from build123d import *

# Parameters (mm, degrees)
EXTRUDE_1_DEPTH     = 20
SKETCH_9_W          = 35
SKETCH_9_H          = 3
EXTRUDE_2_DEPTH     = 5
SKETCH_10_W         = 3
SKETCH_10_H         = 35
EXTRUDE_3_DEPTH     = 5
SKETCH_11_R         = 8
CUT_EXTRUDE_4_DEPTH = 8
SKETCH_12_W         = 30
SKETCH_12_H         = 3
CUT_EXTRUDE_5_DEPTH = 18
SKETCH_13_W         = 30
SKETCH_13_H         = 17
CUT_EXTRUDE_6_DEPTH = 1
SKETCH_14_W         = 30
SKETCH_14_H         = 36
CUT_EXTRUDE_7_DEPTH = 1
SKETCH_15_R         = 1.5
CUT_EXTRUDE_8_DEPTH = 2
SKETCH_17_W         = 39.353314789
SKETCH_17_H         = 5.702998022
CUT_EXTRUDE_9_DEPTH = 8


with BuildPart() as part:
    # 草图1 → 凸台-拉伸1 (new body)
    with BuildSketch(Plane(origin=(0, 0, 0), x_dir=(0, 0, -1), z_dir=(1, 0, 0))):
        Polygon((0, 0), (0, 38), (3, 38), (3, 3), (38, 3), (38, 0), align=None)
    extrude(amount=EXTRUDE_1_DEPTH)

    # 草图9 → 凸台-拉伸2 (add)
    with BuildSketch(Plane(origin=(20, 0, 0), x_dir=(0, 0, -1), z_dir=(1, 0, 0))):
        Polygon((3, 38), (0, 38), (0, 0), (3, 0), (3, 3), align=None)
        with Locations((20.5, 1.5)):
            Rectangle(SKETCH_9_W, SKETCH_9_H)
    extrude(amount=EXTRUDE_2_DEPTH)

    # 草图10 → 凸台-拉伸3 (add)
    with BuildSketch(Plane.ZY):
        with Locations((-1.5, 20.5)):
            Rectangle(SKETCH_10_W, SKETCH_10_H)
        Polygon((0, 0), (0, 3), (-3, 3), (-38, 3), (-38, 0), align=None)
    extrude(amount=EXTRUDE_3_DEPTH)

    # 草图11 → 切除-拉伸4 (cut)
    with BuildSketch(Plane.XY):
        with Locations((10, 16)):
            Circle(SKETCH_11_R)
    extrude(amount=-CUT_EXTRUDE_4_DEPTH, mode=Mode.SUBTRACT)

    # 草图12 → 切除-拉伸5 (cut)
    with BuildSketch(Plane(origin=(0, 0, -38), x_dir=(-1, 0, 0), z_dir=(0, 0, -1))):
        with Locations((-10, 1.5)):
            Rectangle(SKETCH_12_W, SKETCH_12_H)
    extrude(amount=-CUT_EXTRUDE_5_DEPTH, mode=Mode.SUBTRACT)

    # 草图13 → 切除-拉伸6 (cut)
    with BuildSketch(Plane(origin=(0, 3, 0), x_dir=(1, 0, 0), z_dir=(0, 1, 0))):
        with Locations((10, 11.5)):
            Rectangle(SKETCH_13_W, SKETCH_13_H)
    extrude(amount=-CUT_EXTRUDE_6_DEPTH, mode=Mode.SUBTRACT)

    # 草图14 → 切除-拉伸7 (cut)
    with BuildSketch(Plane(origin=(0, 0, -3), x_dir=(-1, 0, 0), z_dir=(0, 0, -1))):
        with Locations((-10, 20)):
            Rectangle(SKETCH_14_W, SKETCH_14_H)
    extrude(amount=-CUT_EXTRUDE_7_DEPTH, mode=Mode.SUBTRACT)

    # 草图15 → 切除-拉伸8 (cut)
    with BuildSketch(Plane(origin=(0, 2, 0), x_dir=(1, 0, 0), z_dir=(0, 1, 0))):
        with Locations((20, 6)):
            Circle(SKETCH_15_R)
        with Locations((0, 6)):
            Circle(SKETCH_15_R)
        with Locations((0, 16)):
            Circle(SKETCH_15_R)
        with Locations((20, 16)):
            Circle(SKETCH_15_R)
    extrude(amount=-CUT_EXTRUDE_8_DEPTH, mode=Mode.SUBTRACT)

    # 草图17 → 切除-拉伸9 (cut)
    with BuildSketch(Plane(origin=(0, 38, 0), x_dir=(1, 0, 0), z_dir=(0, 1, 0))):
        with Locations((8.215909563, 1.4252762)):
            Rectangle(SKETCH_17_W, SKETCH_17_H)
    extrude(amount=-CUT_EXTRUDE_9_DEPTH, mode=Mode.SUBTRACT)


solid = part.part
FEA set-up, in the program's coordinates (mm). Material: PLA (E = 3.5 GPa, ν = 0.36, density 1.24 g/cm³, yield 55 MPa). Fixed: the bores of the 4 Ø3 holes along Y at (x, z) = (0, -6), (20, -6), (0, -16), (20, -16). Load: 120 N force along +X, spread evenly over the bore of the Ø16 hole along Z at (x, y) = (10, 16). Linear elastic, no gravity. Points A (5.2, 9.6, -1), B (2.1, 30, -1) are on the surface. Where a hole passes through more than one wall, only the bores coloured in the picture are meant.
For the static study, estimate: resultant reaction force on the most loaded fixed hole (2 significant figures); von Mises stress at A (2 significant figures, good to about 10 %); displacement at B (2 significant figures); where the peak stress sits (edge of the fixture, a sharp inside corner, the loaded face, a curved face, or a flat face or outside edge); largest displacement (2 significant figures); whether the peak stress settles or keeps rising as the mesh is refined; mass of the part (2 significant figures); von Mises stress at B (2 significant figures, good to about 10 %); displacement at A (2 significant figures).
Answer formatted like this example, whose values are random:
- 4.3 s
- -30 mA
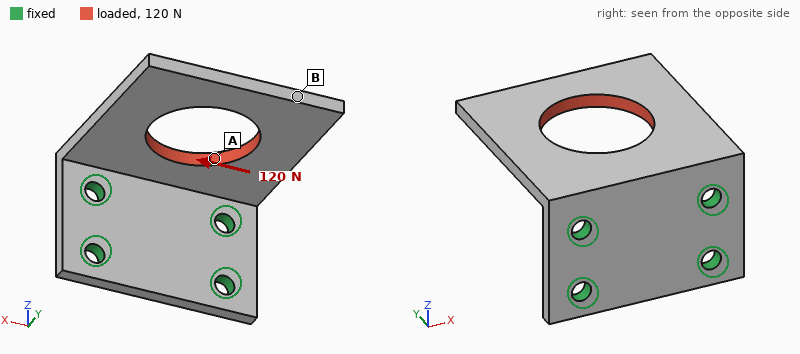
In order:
- 110 N
- 15 MPa
- 0.39 mm
- edge of the fixture
- 0.48 mm
- keeps rising
- 3.0 g
- 4.3 MPa
- 0.12 mm
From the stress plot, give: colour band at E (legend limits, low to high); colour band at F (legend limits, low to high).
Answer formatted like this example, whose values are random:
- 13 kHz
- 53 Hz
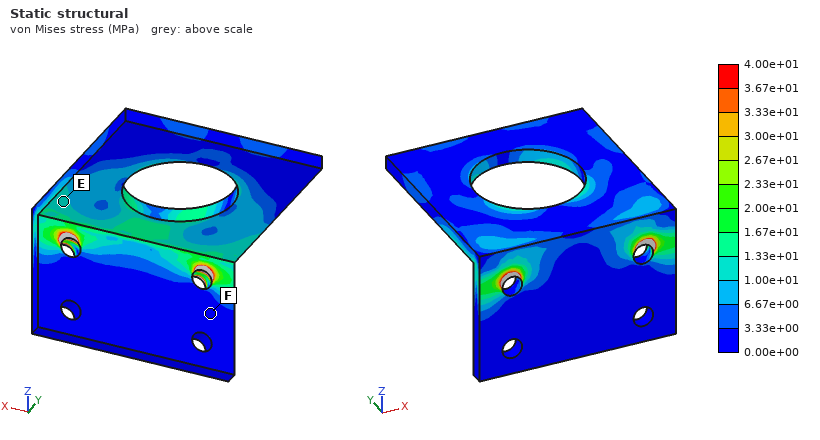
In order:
- 1.00e+01 to 1.33e+01 MPa
- 0.00e+00 to 3.33e+00 MPa
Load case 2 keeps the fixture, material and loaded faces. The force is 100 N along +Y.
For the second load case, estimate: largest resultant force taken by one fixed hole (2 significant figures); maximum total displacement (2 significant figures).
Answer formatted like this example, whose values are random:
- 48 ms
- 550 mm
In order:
- 55 N
- 0.46 mm
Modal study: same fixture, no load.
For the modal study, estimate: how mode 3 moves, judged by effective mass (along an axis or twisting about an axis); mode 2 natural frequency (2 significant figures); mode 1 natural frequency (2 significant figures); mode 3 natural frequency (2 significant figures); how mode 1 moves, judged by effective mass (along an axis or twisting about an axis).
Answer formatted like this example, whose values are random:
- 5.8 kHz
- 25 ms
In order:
- along X
- 1200 Hz
- 520 Hz
- 2600 Hz
- along Z
